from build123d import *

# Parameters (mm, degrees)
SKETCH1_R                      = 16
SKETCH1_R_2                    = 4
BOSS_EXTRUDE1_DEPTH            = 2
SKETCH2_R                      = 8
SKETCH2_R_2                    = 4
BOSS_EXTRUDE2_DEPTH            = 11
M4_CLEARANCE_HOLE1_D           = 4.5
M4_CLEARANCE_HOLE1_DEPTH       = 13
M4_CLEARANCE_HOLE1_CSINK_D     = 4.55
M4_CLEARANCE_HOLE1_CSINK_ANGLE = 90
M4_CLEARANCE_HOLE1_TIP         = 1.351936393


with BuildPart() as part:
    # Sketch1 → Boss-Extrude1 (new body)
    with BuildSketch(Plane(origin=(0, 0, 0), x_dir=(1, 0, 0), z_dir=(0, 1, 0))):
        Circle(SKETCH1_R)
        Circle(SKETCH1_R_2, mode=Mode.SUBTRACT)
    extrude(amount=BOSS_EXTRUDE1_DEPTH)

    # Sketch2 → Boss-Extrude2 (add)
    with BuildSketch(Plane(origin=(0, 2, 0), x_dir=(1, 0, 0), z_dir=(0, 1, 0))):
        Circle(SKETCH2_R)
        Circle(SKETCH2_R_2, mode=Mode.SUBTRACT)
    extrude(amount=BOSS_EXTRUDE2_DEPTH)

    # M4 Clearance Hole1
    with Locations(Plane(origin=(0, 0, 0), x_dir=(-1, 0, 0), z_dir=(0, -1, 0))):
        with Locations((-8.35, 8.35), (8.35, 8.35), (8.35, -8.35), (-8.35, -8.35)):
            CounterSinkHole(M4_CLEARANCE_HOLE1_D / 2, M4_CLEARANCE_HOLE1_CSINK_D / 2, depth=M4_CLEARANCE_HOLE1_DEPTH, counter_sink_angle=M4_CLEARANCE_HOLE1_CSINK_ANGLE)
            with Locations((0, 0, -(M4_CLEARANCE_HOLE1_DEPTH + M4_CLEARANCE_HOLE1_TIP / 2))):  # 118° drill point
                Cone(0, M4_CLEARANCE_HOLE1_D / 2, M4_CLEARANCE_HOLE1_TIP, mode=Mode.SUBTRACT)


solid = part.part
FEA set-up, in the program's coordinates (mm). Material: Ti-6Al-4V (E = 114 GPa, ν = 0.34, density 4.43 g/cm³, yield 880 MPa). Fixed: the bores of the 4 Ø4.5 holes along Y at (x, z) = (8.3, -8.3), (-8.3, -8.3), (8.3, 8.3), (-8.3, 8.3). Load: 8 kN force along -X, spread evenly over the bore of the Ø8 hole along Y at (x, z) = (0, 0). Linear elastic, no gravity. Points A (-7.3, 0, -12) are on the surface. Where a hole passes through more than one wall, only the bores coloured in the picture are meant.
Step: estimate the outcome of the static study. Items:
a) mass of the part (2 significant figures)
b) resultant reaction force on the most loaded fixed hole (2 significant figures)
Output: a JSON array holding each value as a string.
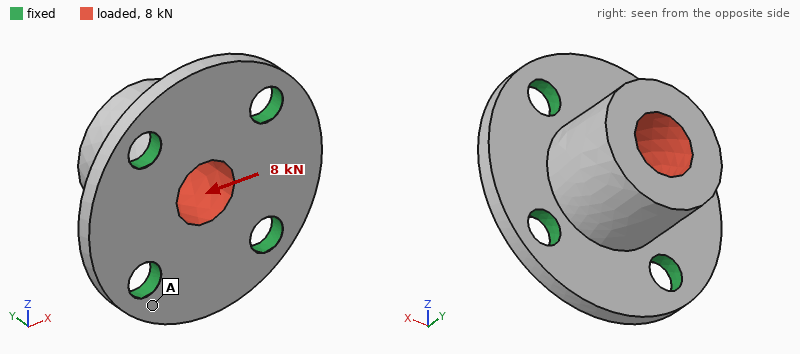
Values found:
["13 g", "2.6 kN"]
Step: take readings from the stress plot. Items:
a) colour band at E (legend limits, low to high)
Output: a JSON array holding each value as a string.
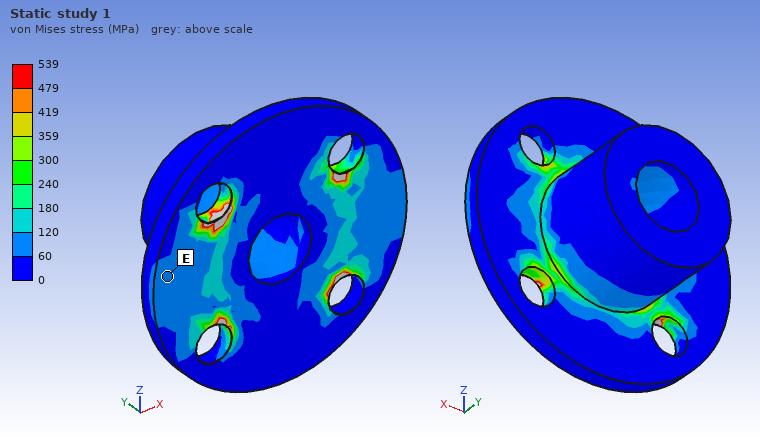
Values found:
["60 to 120 MPa"]
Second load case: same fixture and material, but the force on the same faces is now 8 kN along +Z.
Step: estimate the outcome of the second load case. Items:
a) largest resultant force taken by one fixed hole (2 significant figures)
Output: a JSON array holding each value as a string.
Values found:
["2.6 kN"]
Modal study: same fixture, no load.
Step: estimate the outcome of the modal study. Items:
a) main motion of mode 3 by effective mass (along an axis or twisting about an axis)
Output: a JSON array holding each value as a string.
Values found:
["along Y"]
